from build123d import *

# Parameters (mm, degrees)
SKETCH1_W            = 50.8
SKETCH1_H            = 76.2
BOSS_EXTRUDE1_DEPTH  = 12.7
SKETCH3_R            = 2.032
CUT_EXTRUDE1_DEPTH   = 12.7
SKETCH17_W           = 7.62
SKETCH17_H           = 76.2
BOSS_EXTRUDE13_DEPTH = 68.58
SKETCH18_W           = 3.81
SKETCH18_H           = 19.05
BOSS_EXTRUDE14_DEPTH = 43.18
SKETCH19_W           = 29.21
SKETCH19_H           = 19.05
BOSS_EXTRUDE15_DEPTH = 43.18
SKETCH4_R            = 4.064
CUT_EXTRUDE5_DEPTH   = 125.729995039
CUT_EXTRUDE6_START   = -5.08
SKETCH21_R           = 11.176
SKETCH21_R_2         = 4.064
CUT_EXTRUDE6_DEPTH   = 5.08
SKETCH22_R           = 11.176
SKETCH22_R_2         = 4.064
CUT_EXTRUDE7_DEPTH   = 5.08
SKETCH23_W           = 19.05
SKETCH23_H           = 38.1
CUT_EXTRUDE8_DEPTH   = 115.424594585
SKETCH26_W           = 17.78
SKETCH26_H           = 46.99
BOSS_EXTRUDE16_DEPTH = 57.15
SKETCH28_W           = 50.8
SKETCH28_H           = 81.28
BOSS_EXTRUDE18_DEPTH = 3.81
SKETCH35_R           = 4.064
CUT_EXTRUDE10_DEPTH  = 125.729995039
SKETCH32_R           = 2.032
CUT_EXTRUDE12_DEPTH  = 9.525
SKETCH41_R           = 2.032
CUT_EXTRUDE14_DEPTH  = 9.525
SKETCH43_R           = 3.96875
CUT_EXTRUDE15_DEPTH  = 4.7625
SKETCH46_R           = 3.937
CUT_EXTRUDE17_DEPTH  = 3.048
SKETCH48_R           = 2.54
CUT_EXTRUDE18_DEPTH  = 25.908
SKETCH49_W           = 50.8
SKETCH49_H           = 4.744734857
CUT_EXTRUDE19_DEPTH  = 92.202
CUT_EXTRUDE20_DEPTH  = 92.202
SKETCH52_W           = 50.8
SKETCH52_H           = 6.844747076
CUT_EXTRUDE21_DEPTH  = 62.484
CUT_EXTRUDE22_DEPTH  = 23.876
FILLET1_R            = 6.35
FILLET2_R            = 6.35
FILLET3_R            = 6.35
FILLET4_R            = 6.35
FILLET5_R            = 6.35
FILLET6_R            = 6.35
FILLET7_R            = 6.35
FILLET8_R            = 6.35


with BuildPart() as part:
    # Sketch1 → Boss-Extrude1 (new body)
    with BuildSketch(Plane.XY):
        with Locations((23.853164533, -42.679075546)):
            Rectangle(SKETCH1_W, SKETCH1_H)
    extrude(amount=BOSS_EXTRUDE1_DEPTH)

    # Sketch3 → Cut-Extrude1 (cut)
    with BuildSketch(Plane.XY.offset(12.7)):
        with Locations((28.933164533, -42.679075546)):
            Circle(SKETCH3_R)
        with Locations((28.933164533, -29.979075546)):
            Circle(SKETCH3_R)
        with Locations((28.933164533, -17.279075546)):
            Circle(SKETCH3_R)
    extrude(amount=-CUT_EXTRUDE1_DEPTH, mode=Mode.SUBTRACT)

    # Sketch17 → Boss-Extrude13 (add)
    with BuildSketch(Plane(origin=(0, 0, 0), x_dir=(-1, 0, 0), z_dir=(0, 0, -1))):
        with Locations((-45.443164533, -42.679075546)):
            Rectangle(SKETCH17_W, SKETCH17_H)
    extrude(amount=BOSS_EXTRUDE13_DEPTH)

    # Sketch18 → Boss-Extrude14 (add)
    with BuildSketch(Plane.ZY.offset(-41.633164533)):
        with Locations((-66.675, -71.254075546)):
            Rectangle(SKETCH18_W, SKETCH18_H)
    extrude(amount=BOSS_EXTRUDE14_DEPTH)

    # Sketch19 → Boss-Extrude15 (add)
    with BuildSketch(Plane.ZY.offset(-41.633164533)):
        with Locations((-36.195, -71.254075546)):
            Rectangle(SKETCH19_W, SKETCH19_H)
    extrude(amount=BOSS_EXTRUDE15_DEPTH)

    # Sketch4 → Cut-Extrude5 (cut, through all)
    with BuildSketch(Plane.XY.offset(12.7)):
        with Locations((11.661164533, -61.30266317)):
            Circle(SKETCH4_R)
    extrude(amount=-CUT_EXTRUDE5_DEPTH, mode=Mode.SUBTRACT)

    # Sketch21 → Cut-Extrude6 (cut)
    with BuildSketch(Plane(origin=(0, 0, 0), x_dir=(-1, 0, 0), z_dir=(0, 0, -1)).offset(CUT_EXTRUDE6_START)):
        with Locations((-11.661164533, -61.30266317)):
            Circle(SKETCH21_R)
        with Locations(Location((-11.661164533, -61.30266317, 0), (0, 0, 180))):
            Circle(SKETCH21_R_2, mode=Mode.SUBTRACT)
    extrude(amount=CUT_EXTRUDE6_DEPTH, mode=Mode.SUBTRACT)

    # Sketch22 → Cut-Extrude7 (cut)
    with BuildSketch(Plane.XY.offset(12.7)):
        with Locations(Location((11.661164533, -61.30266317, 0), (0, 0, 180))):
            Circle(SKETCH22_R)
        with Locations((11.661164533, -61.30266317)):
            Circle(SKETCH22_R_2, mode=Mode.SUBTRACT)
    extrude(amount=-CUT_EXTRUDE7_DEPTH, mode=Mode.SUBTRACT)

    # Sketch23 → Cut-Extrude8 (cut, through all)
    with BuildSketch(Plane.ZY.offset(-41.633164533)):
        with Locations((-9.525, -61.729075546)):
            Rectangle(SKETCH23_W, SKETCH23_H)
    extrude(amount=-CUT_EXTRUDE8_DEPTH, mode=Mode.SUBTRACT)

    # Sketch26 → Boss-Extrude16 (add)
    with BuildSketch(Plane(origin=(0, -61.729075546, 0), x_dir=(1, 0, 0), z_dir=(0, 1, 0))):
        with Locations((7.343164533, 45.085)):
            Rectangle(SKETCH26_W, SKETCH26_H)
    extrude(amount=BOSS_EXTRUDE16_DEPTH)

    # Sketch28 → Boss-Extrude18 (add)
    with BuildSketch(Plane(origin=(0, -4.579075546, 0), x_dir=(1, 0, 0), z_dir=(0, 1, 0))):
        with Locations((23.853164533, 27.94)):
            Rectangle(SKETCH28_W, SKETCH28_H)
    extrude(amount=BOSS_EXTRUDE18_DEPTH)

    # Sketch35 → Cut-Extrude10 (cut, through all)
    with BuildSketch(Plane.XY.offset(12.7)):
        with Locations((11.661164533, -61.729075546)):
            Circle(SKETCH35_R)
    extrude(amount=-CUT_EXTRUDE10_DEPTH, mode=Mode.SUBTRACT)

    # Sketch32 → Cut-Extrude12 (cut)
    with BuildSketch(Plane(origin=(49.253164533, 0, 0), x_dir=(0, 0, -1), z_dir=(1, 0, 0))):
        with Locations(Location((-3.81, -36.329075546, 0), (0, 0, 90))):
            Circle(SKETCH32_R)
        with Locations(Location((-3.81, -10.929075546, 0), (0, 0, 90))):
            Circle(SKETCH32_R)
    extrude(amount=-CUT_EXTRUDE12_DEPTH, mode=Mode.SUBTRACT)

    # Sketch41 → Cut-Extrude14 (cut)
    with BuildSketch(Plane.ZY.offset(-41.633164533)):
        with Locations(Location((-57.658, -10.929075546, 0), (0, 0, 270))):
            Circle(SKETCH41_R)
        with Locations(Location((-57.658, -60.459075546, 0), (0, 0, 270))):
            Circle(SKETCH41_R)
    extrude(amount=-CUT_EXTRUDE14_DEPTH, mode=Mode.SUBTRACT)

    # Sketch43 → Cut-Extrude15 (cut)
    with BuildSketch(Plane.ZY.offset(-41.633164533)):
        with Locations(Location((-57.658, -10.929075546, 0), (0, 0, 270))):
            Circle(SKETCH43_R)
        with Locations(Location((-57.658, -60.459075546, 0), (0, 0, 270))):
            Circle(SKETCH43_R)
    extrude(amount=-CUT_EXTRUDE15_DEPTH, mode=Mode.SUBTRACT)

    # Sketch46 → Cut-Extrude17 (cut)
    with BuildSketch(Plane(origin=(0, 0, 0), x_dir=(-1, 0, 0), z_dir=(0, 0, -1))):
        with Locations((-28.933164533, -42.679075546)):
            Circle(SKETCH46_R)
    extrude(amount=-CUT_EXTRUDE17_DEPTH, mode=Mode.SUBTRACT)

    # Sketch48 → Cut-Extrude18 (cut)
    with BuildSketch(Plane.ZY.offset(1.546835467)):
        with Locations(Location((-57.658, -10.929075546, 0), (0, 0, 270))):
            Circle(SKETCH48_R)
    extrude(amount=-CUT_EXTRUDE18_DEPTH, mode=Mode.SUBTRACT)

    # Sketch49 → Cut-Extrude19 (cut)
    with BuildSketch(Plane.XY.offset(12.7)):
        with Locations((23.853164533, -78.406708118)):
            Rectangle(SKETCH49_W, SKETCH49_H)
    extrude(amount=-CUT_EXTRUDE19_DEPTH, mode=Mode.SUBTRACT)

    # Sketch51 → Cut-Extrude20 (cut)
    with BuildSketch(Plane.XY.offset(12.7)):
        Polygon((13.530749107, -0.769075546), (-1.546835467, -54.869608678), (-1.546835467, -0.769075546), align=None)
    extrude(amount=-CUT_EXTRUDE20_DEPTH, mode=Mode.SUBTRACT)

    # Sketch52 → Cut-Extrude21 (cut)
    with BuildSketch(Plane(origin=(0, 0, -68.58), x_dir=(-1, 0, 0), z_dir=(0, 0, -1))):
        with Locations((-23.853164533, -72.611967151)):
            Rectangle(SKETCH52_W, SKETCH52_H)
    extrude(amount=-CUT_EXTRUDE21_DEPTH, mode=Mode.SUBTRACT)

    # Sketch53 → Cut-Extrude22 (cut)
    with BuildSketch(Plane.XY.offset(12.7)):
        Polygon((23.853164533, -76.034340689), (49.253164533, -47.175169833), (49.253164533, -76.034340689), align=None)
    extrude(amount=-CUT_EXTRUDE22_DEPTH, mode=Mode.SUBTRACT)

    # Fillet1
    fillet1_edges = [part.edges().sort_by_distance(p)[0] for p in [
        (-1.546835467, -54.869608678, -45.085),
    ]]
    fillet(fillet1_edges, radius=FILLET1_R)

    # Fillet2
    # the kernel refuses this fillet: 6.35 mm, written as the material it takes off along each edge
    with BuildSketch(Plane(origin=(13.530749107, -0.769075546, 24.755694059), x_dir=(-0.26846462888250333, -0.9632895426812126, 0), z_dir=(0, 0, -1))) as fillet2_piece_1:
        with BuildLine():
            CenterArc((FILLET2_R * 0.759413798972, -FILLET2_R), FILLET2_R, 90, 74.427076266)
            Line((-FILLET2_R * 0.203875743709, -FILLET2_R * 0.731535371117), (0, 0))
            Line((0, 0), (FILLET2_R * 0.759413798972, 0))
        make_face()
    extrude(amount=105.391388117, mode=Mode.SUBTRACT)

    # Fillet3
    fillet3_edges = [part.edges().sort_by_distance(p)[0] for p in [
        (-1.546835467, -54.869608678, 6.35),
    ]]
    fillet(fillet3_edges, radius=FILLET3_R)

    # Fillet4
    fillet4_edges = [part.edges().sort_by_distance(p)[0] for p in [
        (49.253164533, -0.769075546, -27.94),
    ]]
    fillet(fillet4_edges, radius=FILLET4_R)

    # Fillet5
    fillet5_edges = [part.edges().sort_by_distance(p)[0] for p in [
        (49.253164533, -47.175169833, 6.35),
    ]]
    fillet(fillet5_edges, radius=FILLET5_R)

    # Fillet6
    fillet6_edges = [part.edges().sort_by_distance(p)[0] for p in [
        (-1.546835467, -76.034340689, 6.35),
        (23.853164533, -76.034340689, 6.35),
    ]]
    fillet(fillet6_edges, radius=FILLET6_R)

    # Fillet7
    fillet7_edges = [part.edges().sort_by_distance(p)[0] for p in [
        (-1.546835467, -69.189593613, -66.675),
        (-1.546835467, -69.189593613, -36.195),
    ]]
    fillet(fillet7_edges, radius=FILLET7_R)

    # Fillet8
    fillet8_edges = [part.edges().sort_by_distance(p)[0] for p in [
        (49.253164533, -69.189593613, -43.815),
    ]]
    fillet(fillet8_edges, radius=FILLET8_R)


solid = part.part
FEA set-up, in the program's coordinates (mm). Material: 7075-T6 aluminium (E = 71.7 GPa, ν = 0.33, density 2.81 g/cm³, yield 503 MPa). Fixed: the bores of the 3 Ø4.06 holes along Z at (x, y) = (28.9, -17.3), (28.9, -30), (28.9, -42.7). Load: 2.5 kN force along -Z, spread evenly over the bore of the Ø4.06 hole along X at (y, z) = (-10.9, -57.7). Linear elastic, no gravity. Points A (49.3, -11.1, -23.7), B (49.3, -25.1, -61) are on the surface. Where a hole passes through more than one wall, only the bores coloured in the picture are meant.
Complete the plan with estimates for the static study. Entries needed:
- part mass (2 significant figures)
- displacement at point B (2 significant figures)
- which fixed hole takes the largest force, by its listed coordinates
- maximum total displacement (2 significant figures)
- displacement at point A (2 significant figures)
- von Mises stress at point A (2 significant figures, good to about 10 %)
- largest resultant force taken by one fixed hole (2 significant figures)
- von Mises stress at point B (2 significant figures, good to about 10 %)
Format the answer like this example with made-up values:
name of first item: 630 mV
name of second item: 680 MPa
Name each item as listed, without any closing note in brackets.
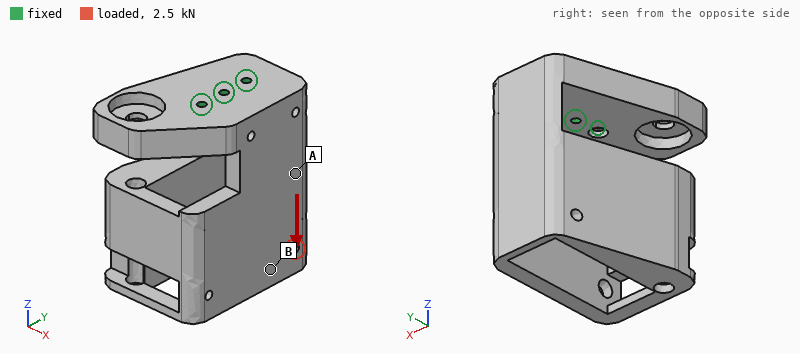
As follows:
part mass: 310 g
displacement at point B: 0.11 mm
which fixed hole takes the largest force, by its listed coordinates: (28.9, -17.3)
maximum total displacement: 0.16 mm
displacement at point A: 0.052 mm
von Mises stress at point A: 18 MPa
largest resultant force taken by one fixed hole: 2.3 kN
von Mises stress at point B: 6.6 MPa
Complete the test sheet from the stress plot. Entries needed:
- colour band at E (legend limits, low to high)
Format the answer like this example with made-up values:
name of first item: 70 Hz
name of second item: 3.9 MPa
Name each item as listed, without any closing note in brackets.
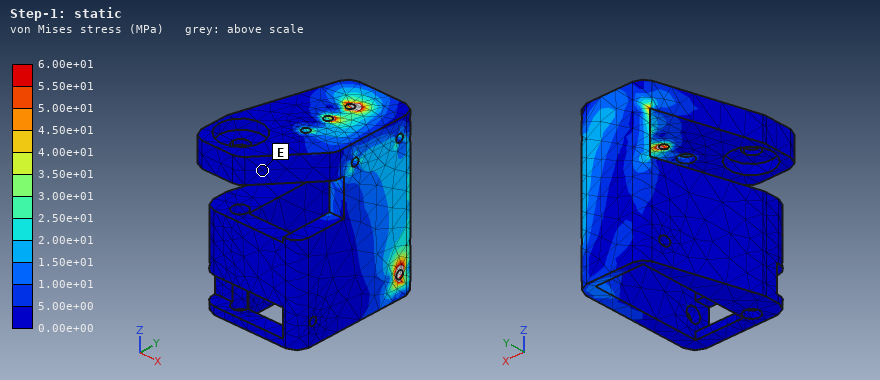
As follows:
colour band at E: 0.00e+00 to 5.00e+00 MPa
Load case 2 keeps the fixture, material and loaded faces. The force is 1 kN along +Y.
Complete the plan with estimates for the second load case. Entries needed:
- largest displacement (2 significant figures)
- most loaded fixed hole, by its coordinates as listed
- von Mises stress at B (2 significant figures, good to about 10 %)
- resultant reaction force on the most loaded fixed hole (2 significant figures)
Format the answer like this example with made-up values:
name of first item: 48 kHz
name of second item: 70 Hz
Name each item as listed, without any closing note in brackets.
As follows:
largest displacement: 0.15 mm
most loaded fixed hole, by its coordinates as listed: (28.9, -17.3)
von Mises stress at B: 6.9 MPa
resultant reaction force on the most loaded fixed hole: 2.1 kN
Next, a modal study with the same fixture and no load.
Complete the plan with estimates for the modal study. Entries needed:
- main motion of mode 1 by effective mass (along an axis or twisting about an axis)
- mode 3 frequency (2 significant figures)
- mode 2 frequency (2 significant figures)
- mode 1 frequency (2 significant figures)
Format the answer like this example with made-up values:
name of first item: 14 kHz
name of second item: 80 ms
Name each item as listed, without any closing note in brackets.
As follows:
main motion of mode 1 by effective mass: along X
mode 3 frequency: 2200 Hz
mode 2 frequency: 890 Hz
mode 1 frequency: 730 Hz
